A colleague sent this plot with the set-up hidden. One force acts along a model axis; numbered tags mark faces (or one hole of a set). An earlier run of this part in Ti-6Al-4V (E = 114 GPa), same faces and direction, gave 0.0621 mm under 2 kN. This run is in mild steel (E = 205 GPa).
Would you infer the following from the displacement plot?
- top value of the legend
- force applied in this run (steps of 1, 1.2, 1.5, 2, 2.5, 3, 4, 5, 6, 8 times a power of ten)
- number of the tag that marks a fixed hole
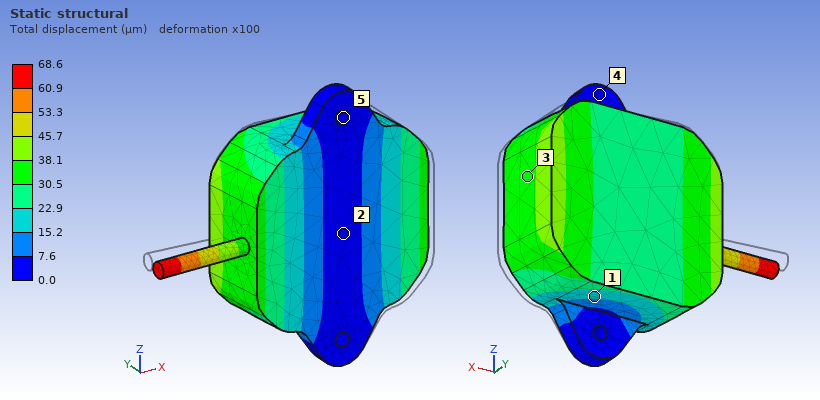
68.6 µm
4 kN
5
